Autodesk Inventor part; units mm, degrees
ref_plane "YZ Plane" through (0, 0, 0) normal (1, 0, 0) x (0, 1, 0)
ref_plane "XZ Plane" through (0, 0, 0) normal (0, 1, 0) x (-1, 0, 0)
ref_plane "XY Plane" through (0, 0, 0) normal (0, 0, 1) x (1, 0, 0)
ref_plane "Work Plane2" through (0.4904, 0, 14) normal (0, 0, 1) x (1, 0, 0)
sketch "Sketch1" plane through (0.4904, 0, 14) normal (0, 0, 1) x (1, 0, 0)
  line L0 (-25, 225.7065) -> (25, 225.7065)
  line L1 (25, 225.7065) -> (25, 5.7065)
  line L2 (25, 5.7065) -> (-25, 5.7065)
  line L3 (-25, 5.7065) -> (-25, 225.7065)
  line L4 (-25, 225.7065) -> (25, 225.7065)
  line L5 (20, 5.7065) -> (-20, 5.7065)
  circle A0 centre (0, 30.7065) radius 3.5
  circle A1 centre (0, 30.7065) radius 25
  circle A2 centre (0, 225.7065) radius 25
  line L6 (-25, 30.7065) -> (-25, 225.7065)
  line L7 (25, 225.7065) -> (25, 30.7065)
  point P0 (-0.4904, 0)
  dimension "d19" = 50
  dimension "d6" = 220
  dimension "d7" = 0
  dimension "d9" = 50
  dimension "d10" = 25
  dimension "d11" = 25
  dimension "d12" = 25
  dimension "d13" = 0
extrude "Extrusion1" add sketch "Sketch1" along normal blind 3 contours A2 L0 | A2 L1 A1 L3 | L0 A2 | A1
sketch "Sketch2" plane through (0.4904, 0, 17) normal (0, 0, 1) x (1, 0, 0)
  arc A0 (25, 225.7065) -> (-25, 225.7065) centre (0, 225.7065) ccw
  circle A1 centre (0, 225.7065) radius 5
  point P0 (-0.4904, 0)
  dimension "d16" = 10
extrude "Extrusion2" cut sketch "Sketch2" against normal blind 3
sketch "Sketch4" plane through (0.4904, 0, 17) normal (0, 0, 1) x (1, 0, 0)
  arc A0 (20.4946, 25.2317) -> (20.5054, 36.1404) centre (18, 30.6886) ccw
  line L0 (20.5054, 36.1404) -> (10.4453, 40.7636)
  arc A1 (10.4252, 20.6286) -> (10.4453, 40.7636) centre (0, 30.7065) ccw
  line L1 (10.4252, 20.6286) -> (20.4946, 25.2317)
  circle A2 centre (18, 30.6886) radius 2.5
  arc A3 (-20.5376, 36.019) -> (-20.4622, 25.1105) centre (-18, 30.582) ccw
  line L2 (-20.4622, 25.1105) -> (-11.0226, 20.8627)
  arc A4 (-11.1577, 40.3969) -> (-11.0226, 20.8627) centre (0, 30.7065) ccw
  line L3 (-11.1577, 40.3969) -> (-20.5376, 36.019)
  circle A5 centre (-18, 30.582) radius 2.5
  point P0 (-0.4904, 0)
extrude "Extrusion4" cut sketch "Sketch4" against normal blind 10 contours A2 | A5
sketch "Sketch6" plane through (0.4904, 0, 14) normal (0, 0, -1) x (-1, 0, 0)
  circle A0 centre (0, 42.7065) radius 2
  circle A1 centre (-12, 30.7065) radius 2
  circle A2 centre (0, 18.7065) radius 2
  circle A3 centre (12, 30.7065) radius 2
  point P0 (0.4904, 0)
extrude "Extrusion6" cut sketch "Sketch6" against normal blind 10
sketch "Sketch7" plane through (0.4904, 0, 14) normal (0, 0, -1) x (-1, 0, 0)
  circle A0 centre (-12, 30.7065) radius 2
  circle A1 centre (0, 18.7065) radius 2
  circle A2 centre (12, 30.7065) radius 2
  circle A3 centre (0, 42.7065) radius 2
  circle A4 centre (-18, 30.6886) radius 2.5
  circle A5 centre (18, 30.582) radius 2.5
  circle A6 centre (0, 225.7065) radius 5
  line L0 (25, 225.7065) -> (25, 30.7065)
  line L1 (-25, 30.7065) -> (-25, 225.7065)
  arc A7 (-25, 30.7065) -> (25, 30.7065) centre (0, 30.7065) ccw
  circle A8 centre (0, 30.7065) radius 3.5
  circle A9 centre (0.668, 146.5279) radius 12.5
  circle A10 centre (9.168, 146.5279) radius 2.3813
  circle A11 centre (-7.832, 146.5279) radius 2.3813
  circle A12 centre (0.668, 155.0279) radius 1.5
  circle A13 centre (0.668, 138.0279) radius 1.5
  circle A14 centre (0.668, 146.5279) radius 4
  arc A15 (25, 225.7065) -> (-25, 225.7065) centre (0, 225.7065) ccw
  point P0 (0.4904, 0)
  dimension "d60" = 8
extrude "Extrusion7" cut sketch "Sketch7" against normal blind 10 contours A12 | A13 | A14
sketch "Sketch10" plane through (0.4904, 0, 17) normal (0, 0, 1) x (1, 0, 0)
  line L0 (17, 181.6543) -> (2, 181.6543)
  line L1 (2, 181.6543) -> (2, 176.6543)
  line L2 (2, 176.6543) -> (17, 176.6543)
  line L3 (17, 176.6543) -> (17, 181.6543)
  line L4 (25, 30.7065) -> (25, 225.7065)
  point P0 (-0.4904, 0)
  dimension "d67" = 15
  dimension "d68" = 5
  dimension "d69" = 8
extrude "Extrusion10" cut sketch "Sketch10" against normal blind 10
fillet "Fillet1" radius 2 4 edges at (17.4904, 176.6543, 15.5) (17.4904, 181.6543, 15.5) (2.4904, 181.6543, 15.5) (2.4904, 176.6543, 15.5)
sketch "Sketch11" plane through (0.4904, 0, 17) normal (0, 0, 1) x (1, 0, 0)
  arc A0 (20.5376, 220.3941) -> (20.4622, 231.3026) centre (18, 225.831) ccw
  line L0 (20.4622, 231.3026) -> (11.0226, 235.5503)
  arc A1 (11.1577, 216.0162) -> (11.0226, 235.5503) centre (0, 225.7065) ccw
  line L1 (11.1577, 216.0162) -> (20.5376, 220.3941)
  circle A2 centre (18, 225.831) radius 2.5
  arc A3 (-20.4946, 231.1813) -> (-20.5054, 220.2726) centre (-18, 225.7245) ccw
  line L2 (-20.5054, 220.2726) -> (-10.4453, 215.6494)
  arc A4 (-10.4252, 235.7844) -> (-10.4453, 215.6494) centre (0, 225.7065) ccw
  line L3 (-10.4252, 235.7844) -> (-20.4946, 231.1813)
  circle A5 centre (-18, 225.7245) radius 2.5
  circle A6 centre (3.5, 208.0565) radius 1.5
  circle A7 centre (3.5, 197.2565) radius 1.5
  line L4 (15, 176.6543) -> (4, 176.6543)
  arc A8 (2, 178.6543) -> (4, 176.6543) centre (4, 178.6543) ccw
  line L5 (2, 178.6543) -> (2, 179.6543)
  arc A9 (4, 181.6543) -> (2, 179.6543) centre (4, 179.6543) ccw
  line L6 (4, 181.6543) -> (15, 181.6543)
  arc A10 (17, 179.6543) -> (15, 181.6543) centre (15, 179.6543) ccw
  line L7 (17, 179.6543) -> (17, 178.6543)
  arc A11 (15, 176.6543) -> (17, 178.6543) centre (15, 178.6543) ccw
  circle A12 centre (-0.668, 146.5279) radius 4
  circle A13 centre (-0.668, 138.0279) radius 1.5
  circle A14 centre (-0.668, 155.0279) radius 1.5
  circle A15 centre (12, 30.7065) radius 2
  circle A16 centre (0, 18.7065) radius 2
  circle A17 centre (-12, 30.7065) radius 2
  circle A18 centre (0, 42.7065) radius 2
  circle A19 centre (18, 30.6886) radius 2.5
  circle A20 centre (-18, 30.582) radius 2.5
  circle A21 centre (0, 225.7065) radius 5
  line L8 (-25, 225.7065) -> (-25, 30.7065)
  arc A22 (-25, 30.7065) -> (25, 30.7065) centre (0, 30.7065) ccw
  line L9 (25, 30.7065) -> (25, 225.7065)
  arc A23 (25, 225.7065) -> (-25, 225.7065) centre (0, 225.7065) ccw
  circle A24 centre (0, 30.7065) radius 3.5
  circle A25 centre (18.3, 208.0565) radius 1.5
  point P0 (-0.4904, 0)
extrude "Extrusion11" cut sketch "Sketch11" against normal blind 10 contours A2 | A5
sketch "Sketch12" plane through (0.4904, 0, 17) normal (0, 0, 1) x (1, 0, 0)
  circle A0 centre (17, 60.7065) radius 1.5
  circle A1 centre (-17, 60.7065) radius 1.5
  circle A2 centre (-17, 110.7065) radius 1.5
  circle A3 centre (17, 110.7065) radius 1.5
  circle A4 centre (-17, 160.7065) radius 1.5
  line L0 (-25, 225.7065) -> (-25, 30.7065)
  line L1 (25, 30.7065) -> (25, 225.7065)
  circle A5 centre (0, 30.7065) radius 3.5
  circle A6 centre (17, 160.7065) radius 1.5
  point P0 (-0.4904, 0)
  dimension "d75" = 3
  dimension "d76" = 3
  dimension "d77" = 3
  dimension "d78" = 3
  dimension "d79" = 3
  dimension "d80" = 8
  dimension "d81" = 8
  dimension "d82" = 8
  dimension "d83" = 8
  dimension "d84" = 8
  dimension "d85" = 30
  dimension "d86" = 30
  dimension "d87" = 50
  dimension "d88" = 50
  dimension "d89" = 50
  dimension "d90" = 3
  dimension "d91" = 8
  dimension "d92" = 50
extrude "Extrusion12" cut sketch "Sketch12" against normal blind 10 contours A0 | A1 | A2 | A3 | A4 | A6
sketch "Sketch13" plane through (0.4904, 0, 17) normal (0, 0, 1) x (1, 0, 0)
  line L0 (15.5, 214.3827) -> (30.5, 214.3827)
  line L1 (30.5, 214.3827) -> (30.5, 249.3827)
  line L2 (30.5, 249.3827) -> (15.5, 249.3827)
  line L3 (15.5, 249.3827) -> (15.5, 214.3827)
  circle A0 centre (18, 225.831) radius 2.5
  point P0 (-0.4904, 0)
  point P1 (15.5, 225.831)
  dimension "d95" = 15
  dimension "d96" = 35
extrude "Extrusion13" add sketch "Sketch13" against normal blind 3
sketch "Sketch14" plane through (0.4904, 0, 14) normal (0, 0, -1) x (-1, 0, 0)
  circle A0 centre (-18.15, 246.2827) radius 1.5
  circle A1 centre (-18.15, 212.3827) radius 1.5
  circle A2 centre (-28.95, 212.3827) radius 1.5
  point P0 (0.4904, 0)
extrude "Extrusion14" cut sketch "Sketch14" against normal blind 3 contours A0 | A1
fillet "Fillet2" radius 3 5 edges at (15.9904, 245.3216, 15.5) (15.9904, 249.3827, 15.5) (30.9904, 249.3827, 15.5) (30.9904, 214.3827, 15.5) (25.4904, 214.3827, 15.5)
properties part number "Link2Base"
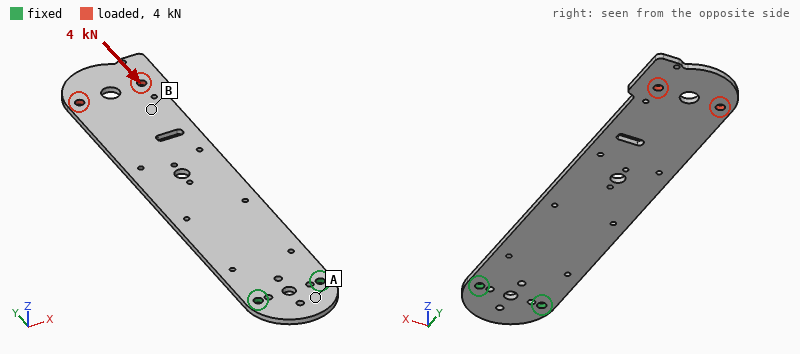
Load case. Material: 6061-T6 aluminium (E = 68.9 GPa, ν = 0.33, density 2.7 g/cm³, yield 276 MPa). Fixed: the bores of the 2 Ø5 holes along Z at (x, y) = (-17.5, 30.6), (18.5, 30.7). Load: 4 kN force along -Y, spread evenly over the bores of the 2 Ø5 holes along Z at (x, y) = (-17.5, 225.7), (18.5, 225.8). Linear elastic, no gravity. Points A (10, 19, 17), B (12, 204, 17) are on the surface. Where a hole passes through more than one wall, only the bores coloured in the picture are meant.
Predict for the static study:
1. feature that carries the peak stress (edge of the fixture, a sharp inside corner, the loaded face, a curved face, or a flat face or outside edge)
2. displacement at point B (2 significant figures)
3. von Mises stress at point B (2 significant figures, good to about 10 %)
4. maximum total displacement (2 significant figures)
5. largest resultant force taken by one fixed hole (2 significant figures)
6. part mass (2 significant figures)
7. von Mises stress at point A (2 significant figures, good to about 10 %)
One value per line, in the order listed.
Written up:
a curved face
78 µm
23 MPa
94 µm
2.0 kN
94 g
8.7 MPa
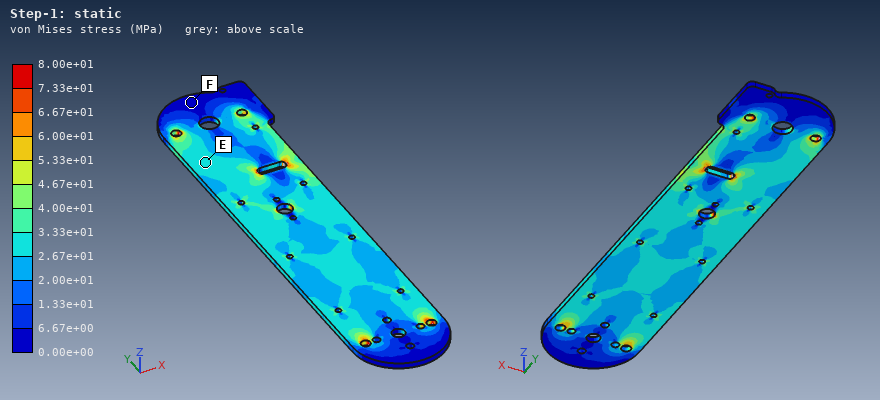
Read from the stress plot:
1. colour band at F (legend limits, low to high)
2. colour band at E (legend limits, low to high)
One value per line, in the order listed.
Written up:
0.00e+00 to 6.67e+00 MPa
2.67e+01 to 3.33e+01 MPa
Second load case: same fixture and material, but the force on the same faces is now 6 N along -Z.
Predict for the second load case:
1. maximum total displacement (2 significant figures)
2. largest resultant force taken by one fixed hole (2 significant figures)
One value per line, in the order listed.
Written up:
2.4 mm
3.1 N
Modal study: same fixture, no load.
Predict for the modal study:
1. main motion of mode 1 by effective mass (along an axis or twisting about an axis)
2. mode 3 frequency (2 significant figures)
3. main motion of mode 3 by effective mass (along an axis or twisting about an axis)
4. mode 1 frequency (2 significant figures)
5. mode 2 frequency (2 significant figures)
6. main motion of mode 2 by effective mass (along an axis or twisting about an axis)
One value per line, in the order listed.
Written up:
along Z
430 Hz
twisting about Y
51 Hz
310 Hz
along Z
